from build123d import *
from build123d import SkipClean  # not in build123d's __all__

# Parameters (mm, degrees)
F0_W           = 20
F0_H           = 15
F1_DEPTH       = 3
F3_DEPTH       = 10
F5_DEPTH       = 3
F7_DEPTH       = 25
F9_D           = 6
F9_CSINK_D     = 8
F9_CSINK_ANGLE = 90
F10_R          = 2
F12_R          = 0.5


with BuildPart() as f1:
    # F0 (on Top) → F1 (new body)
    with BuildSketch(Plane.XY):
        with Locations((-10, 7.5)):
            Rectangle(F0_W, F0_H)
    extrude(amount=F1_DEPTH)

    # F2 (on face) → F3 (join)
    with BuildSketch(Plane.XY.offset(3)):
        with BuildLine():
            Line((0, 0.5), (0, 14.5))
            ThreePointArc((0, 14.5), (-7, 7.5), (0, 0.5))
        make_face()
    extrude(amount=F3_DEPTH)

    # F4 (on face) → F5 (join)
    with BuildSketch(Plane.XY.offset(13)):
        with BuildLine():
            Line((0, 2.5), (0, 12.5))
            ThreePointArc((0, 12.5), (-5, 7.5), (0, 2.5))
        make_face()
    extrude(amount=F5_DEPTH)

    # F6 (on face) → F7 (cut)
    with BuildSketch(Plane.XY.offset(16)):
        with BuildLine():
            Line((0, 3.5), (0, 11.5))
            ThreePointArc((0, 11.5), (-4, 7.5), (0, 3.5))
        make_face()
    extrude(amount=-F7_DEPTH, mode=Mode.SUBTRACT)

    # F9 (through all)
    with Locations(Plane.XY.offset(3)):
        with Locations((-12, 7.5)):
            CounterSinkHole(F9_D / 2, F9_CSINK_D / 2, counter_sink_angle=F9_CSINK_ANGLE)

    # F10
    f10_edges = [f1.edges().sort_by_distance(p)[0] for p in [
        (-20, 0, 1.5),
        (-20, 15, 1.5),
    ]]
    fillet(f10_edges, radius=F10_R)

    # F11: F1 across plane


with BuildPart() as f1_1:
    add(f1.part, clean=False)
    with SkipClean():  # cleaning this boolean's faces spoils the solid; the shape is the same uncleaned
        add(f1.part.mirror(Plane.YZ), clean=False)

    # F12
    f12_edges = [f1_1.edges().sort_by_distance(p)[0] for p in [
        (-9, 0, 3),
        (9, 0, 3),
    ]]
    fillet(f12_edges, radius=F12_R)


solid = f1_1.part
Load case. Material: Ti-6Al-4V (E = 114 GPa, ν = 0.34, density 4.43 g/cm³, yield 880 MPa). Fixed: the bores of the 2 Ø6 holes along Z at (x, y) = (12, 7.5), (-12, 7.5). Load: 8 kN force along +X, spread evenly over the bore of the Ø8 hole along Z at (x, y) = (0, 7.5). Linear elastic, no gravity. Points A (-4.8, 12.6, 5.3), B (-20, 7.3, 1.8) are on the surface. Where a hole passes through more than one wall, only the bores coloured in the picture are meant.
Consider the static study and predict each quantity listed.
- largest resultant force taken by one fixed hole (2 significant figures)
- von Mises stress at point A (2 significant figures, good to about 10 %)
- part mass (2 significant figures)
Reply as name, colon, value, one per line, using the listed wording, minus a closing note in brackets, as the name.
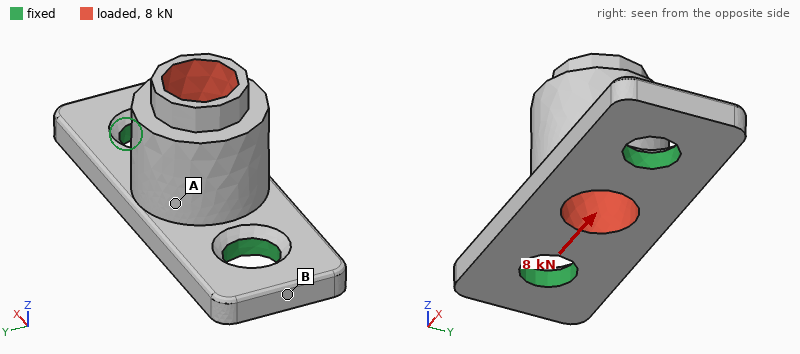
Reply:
largest resultant force taken by one fixed hole: 5.1 kN
von Mises stress at point A: 110 MPa
part mass: 11 g
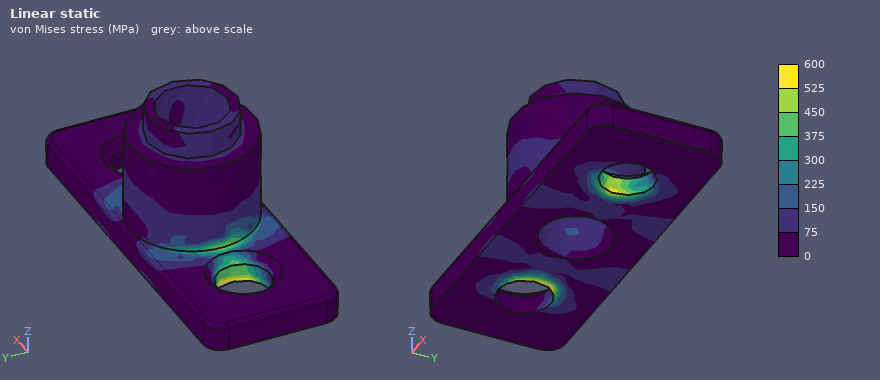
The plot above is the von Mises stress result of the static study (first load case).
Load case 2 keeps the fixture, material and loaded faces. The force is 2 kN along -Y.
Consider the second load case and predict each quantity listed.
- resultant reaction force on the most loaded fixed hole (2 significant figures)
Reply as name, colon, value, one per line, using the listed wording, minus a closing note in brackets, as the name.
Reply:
resultant reaction force on the most loaded fixed hole: 1.0 kN
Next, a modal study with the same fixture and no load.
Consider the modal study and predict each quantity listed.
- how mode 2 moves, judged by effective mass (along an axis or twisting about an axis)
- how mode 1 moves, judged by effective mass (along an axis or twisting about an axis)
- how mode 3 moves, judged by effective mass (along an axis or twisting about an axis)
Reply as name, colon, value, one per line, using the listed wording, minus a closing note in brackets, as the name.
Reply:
how mode 2 moves, judged by effective mass: along Z
how mode 1 moves, judged by effective mass: along Y
how mode 3 moves, judged by effective mass: along X
